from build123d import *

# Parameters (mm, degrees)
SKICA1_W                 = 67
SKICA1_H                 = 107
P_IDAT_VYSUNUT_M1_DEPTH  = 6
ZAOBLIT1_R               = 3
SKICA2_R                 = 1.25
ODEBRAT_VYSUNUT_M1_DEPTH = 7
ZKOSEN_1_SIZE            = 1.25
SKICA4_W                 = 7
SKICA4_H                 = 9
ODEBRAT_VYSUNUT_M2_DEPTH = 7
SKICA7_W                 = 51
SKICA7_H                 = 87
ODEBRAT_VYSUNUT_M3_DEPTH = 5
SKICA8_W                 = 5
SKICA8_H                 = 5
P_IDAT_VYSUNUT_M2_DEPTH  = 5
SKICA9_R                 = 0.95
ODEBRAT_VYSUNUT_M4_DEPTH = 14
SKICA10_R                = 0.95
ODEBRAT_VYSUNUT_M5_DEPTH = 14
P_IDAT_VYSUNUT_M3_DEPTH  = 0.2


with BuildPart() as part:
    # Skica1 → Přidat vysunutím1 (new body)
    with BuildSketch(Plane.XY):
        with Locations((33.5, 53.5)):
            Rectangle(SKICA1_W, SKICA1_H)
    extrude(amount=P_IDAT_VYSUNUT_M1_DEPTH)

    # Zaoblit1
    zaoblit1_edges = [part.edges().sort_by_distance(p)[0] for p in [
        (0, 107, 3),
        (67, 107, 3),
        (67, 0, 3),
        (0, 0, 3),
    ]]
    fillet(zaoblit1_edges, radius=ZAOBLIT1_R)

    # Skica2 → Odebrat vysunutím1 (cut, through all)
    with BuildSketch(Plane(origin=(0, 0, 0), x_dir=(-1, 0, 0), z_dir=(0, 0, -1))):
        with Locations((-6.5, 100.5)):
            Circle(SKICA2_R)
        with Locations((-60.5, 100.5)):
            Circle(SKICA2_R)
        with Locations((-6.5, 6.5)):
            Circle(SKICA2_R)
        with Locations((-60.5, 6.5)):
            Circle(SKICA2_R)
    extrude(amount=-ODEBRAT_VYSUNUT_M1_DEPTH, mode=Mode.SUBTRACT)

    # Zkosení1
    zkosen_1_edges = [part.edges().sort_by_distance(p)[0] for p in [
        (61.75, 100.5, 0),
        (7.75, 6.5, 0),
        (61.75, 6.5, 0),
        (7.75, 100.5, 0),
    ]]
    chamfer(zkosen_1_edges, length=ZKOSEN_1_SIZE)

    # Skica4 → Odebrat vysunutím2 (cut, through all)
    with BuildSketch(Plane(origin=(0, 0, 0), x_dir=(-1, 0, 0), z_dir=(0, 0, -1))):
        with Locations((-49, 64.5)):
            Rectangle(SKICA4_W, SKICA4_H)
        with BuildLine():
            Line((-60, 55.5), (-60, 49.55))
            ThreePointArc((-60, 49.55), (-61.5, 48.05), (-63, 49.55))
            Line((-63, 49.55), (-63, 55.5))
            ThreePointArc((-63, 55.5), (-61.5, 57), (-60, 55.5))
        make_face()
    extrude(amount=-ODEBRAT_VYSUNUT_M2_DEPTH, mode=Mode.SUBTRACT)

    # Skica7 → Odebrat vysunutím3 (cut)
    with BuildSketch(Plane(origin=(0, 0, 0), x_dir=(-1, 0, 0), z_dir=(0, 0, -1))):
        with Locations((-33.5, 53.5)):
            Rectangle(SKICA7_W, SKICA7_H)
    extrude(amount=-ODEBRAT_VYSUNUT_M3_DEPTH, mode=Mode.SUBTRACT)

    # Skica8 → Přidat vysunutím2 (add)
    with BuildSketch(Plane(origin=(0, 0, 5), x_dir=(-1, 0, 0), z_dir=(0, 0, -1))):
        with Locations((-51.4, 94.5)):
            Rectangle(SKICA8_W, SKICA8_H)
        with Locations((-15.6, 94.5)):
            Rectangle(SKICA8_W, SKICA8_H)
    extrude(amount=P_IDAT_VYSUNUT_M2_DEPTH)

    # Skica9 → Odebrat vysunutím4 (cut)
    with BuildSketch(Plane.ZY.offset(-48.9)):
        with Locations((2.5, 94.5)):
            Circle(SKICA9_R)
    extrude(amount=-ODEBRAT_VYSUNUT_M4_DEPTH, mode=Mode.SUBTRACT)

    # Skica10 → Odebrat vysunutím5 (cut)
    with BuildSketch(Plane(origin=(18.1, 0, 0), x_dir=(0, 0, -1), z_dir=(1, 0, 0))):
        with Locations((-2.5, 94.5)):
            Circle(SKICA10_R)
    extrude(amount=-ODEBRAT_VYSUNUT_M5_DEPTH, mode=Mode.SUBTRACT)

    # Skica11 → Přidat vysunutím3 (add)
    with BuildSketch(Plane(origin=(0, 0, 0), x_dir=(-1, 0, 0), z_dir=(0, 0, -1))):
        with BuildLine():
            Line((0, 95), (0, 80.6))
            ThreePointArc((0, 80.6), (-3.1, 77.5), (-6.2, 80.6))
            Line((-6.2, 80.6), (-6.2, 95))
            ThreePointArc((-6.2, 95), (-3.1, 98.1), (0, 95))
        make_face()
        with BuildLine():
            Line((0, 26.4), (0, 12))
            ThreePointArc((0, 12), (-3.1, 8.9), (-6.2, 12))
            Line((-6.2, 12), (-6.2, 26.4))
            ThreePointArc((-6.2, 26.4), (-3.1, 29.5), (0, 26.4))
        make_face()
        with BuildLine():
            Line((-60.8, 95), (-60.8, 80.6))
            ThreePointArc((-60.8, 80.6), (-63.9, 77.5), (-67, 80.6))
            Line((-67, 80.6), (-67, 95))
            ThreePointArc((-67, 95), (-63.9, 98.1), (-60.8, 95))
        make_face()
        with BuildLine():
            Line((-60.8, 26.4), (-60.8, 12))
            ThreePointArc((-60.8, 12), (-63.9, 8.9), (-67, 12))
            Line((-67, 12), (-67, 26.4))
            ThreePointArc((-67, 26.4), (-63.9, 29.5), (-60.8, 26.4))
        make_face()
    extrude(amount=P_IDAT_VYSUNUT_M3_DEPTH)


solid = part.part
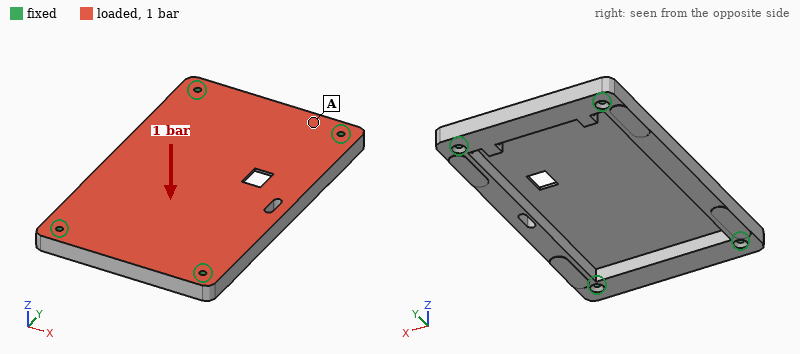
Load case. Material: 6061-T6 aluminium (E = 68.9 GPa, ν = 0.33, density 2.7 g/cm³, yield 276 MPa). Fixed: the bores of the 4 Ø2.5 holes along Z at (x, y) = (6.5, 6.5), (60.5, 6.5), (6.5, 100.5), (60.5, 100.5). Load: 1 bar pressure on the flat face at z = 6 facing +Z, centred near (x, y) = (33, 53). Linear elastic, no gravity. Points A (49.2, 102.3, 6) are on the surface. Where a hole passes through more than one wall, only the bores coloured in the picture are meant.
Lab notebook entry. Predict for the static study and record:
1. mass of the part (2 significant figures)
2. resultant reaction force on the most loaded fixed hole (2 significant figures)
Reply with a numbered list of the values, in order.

1. 56 g
2. 200 N
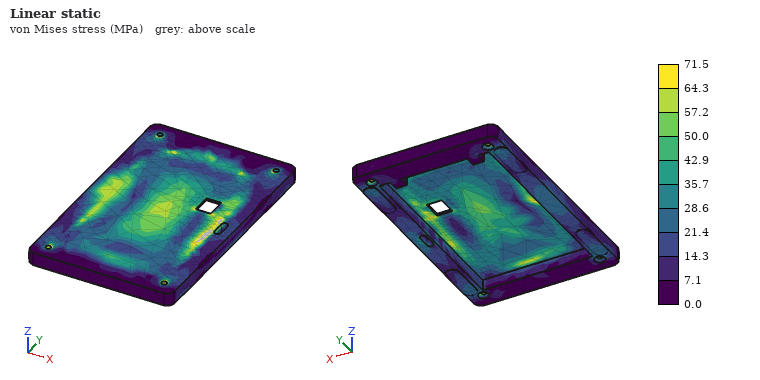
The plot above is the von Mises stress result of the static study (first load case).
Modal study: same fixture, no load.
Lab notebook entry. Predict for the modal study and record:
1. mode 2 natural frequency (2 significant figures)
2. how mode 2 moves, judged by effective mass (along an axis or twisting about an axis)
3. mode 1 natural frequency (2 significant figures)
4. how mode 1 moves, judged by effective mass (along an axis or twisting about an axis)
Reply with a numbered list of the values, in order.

1. 3200 Hz
2. twisting about Y
3. 2100 Hz
4. along Z
